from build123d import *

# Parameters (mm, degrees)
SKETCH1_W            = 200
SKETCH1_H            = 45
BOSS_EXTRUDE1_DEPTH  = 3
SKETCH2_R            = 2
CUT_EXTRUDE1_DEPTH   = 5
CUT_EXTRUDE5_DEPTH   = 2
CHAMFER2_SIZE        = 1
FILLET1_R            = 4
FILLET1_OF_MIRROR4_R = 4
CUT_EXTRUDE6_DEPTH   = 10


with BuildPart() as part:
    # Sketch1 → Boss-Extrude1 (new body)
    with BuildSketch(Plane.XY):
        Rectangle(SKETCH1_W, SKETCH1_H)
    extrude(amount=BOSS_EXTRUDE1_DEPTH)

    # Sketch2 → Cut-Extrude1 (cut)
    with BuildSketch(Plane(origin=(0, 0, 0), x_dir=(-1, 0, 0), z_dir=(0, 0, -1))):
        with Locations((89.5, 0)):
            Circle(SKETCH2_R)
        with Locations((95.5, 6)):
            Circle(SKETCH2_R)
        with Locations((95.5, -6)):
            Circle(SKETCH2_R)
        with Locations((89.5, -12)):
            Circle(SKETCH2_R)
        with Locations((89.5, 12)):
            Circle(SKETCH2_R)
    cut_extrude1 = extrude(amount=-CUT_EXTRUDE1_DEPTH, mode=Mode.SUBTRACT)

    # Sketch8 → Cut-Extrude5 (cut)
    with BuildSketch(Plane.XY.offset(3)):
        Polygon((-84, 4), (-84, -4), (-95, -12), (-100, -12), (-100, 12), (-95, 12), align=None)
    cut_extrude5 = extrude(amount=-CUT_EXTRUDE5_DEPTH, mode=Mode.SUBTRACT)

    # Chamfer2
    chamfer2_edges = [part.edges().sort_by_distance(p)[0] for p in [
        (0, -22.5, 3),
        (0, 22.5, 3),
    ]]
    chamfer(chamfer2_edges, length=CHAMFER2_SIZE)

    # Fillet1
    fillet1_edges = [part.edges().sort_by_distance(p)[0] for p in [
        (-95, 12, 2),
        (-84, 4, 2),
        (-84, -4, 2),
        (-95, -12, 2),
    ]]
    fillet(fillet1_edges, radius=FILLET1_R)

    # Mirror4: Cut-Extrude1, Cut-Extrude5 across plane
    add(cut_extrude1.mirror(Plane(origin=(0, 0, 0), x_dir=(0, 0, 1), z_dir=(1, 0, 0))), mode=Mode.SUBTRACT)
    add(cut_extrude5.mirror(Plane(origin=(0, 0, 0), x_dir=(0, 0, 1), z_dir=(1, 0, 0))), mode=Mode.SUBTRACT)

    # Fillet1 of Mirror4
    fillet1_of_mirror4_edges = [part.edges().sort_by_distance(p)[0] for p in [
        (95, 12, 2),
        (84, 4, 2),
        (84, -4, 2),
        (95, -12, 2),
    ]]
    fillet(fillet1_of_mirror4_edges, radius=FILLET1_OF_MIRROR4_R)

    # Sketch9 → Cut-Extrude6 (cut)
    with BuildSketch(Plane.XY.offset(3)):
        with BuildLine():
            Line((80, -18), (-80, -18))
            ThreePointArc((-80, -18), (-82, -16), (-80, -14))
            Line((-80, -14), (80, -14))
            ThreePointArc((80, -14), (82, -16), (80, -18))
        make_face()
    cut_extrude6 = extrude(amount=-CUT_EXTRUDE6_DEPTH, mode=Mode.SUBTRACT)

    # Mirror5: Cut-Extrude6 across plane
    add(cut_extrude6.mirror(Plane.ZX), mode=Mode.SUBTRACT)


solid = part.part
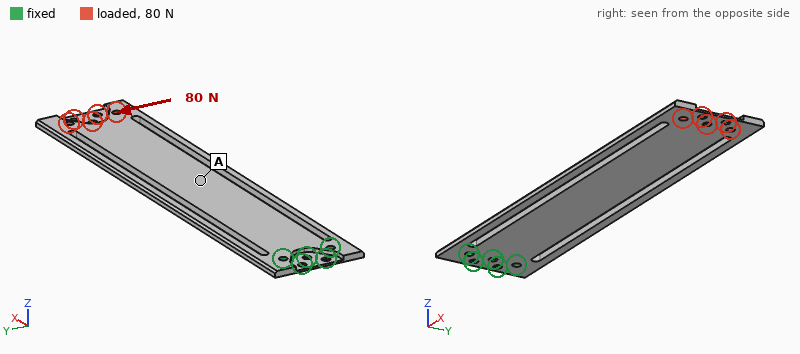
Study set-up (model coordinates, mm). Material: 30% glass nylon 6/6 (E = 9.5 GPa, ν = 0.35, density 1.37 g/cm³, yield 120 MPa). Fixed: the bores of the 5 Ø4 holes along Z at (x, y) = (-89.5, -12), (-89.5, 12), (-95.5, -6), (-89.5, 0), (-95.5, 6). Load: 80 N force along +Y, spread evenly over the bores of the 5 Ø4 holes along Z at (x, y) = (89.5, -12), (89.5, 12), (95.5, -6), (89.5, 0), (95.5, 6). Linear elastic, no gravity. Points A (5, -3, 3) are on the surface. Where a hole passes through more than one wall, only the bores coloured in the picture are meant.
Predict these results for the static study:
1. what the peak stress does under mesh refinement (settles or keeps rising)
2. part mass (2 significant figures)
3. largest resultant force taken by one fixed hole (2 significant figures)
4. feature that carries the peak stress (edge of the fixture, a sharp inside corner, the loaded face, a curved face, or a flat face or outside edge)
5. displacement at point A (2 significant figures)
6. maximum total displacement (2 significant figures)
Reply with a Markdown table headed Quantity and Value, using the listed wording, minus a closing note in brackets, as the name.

| Quantity | Value |
|---|---|
| what the peak stress does under mesh refinement | keeps rising |
| part mass | 29 g |
| largest resultant force taken by one fixed hole | 530 N |
| feature that carries the peak stress | edge of the fixture |
| displacement at point A | 0.63 mm |
| maximum total displacement | 1.7 mm |
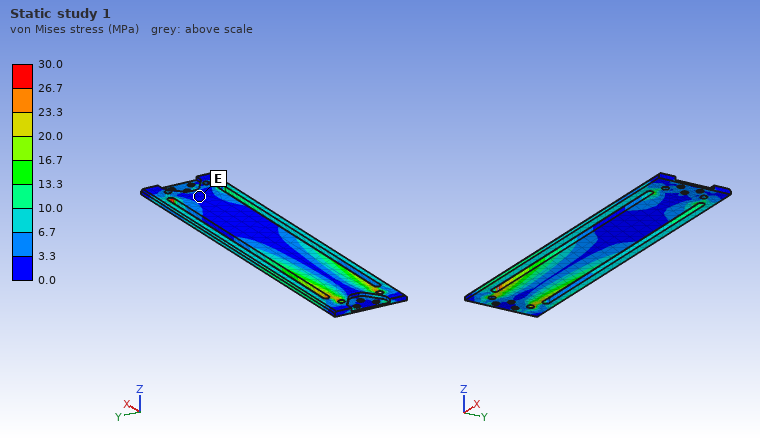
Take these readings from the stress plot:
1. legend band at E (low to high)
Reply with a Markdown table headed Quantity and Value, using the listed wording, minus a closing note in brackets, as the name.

| Quantity | Value |
|---|---|
| legend band at E | 0.0 to 3.3 MPa |
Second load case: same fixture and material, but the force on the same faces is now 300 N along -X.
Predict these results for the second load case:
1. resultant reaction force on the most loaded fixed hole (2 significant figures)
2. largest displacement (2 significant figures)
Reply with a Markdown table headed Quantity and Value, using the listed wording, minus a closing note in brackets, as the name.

| Quantity | Value |
|---|---|
| resultant reaction force on the most loaded fixed hole | 120 N |
| largest displacement | 2.1 mm |
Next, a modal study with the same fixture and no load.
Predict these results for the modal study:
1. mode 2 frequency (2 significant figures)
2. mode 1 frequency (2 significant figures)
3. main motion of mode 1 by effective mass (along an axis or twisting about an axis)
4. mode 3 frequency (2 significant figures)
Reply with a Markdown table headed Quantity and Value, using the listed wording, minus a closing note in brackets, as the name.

| Quantity | Value |
|---|---|
| mode 2 frequency | 230 Hz |
| mode 1 frequency | 36 Hz |
| main motion of mode 1 by effective mass | along Z |
| mode 3 frequency | 230 Hz |
